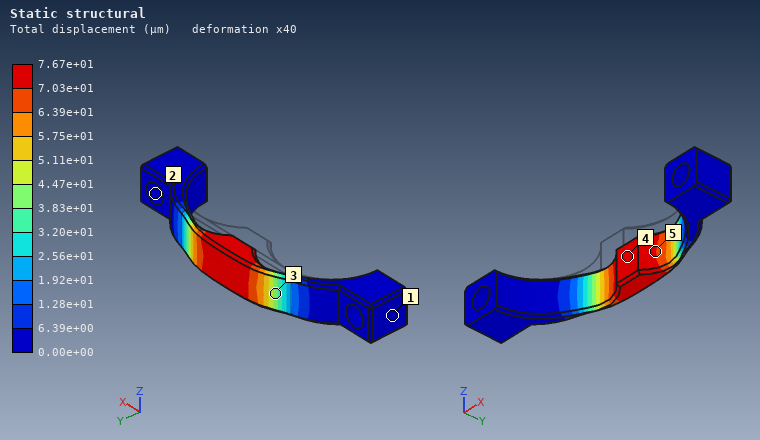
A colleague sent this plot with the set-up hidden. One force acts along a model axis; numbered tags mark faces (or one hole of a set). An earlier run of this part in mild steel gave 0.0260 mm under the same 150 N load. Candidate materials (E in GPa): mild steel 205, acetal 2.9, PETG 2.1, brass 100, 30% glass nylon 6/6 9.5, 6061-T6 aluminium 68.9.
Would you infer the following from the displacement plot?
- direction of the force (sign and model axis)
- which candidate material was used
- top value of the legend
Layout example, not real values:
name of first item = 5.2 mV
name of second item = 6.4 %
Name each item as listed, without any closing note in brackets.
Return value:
direction of the force = +Y
which candidate material was used = 6061-T6 aluminium
top value of the legend = 7.67e+01 µm
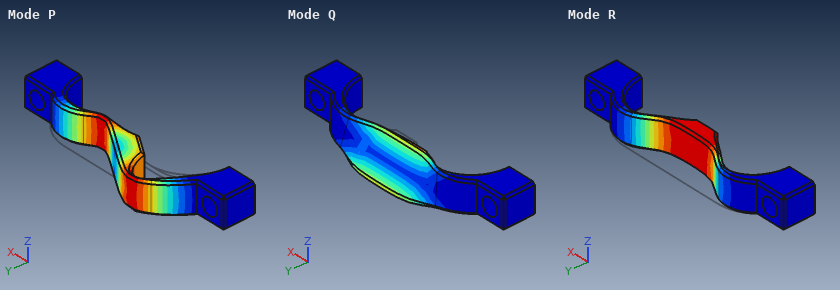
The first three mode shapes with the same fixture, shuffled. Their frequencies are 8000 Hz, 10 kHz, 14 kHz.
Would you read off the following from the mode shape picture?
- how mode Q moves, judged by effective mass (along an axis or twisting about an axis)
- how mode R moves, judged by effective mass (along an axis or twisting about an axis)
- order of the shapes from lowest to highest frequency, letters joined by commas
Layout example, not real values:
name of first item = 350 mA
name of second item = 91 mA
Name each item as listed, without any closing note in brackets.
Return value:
how mode Q moves, judged by effective mass = along Z
how mode R moves, judged by effective mass = along Y
order of the shapes from lowest to highest frequency, letters joined by commas = R, Q, P
